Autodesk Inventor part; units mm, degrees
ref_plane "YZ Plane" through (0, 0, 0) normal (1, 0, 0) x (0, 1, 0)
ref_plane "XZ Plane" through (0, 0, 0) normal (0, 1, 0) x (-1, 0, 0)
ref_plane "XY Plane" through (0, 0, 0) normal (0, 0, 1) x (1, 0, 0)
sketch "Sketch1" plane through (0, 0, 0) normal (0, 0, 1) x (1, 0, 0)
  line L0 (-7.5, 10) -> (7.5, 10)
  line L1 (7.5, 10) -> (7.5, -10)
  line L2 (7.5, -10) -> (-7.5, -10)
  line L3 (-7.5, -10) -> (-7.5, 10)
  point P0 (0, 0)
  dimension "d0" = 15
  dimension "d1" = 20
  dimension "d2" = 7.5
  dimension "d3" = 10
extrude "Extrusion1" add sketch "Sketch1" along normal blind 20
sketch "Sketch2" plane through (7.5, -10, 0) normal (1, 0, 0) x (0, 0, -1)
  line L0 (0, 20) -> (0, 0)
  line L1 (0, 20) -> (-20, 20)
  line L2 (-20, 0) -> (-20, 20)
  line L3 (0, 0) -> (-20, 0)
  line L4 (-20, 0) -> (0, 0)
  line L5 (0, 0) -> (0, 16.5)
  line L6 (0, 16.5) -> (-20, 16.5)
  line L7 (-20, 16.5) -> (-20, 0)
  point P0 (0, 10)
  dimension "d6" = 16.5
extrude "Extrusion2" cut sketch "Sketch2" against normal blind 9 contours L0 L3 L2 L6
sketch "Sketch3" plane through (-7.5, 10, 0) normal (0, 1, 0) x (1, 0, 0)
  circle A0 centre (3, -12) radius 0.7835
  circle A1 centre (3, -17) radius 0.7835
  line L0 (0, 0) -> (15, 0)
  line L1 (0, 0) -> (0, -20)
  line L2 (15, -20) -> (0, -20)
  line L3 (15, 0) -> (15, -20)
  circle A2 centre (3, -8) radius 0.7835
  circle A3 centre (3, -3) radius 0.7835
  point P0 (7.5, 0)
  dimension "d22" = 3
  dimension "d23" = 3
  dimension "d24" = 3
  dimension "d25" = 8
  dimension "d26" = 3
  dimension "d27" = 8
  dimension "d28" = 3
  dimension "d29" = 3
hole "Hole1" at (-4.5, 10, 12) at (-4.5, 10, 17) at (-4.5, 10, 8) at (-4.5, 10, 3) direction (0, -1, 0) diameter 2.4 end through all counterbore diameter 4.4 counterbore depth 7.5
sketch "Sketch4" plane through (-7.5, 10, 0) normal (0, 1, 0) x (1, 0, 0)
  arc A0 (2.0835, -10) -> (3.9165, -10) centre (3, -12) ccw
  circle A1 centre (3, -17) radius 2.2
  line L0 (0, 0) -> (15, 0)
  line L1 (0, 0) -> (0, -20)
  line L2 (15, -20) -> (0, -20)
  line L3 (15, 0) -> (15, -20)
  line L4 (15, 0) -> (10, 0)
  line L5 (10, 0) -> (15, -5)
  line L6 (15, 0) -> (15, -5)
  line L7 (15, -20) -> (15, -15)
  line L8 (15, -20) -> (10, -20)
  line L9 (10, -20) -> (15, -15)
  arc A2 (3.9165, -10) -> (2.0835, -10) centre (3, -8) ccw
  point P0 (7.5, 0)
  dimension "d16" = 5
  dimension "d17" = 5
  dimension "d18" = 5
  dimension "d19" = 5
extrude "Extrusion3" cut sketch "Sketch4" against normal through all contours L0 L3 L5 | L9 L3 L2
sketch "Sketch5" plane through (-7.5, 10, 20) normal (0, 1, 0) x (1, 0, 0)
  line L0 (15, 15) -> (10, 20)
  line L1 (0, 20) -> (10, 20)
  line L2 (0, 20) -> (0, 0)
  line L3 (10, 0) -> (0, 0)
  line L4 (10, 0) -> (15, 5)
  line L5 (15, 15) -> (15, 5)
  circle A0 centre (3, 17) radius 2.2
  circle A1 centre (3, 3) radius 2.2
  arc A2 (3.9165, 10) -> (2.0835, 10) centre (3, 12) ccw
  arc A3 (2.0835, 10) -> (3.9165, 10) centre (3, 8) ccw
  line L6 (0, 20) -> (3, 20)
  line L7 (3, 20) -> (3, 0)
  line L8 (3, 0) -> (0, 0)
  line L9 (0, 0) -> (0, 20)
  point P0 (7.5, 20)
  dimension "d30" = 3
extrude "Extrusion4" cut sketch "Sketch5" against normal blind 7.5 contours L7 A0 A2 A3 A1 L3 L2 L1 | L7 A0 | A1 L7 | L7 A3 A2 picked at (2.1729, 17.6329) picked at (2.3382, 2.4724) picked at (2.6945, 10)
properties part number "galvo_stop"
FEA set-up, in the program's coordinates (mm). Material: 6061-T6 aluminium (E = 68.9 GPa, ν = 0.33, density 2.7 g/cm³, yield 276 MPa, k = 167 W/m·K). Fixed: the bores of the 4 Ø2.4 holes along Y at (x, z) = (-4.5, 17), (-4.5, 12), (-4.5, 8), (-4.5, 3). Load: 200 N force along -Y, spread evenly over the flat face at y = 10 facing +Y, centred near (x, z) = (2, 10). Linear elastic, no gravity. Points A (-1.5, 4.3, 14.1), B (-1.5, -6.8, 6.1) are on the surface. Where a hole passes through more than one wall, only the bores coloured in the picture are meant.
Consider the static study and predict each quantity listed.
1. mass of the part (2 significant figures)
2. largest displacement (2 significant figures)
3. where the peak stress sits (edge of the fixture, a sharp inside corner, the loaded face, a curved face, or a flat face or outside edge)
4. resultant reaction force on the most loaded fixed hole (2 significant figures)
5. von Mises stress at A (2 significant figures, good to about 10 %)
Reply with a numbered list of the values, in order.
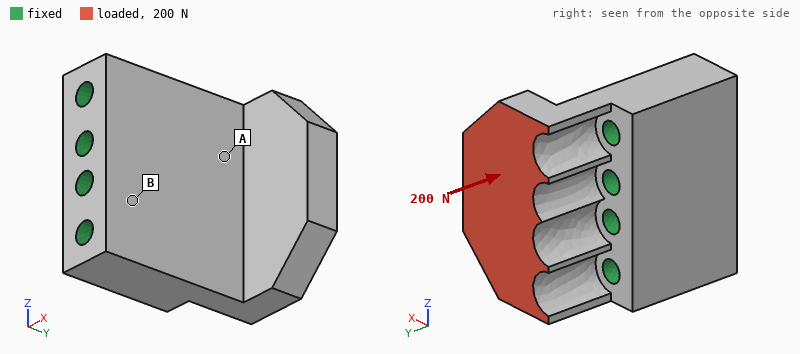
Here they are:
1. 5.5 g
2. 62 µm
3. a curved face
4. 61 N
5. 54 MPa
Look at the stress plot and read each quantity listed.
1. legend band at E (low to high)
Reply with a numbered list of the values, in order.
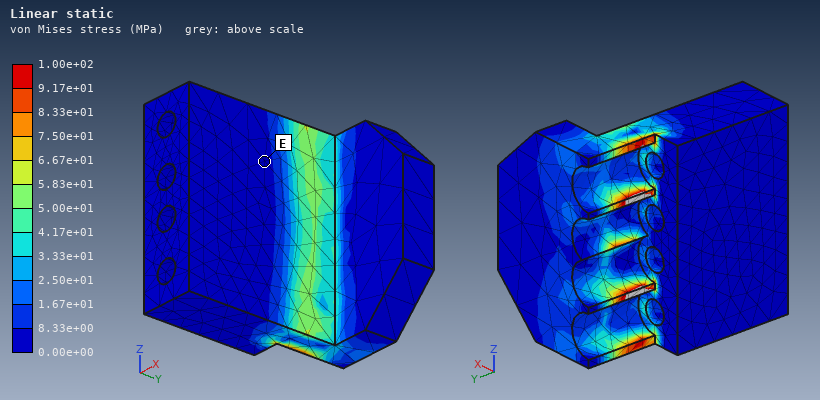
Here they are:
1. 0.00e+00 to 8.33e+00 MPa
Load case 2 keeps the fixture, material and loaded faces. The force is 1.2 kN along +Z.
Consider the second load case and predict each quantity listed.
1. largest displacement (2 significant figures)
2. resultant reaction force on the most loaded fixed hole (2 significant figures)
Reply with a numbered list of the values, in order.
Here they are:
1. 47 µm
2. 800 N
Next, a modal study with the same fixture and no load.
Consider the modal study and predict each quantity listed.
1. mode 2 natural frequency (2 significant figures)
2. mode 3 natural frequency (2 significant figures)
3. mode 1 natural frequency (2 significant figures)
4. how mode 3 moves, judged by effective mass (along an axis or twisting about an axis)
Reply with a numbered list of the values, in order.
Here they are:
1. 16 kHz
2. 25 kHz
3. 7400 Hz
4. along X
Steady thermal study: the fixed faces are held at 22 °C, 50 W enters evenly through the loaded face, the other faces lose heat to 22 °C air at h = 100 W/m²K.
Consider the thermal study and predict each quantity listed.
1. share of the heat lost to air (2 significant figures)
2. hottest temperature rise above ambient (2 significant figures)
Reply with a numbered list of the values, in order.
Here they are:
1. 6.5 %
2. 78 K
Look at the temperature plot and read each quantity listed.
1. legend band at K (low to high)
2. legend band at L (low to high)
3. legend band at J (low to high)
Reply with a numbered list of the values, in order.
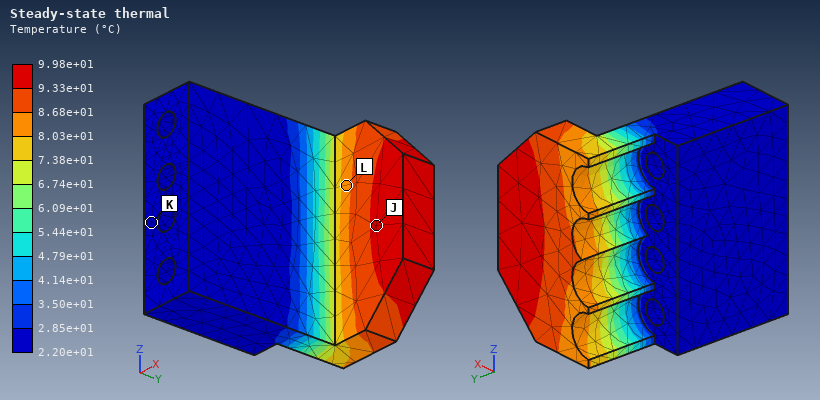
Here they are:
1. 2.20e+01 to 2.85e+01 °C
2. 8.03e+01 to 8.68e+01 °C
3. 9.33e+01 to 9.98e+01 °C
